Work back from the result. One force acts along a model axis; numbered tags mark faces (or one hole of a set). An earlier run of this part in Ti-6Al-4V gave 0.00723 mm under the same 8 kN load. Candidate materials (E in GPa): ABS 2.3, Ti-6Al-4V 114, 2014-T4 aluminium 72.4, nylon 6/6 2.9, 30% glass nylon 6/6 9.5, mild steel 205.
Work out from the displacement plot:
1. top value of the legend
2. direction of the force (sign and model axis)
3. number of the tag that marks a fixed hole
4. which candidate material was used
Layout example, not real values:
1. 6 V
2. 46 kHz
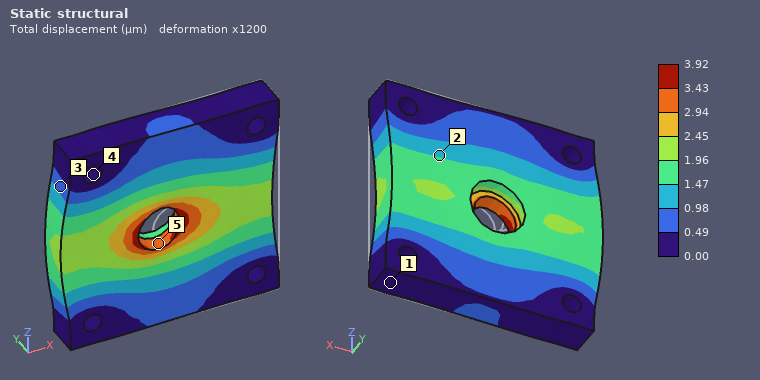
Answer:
1. 3.92 µm
2. -X
3. 4
4. mild steel
